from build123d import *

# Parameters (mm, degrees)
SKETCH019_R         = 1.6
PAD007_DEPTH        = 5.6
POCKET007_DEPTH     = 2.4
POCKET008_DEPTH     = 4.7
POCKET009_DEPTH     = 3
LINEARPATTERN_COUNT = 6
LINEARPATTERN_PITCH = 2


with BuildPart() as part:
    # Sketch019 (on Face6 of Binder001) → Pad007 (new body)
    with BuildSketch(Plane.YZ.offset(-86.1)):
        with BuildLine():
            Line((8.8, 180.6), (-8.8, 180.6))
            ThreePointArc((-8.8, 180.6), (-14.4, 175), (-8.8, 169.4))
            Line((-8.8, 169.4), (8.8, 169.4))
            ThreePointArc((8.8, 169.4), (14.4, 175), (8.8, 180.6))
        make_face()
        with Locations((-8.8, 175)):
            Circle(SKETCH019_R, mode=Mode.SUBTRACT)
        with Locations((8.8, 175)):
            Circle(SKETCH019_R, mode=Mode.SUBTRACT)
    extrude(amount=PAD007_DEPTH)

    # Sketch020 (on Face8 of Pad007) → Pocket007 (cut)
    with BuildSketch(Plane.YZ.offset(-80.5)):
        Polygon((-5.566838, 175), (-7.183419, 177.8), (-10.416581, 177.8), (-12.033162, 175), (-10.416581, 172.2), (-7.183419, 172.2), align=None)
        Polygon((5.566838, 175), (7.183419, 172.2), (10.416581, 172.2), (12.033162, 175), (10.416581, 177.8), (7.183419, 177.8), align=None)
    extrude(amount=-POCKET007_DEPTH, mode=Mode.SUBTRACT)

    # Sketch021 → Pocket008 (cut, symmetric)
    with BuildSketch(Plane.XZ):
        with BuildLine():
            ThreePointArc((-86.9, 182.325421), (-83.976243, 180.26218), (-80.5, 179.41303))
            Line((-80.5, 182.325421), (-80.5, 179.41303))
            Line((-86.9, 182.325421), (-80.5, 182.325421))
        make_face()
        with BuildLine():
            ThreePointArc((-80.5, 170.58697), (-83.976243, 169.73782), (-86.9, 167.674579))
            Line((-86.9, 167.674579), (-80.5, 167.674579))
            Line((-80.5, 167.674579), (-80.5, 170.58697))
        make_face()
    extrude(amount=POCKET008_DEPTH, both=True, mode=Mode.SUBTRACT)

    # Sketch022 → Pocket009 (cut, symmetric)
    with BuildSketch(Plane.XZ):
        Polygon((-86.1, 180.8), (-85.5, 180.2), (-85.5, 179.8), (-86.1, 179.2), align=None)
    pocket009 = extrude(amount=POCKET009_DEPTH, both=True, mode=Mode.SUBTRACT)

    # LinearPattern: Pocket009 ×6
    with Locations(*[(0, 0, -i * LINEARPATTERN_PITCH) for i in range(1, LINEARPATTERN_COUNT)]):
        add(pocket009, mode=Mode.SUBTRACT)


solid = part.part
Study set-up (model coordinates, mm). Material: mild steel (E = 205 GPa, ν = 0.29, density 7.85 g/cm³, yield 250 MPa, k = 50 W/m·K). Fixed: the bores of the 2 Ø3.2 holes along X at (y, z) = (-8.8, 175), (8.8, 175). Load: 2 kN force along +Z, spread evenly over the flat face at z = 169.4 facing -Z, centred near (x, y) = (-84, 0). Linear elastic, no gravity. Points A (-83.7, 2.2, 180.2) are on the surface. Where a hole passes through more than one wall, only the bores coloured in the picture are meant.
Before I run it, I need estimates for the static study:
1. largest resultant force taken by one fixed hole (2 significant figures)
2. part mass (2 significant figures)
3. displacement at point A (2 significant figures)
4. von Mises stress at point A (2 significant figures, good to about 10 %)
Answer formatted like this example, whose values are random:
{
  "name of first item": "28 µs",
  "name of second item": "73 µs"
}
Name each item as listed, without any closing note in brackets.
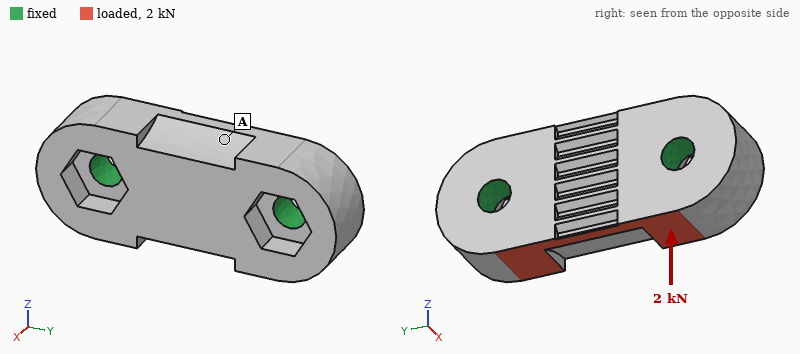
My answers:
{
  "largest resultant force taken by one fixed hole": "1.0 kN",
  "part mass": "11 g",
  "displacement at point A": "1.5 µm",
  "von Mises stress at point A": "21 MPa"
}
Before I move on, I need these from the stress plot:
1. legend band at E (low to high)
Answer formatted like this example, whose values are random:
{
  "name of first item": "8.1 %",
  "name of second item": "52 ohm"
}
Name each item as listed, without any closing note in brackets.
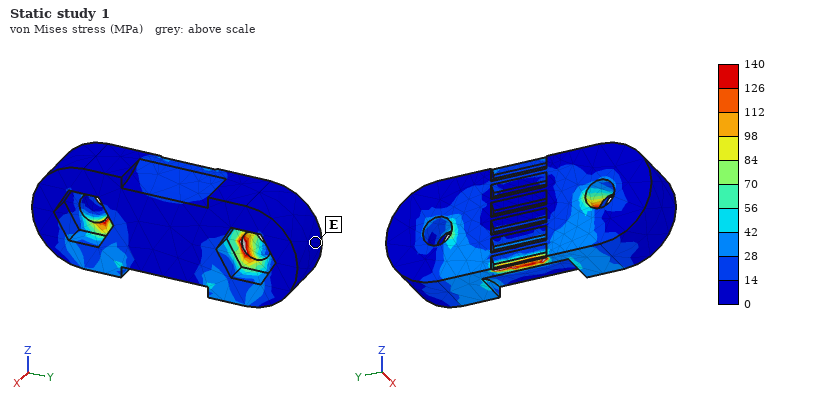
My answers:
{
  "legend band at E": "0 to 14 MPa"
}
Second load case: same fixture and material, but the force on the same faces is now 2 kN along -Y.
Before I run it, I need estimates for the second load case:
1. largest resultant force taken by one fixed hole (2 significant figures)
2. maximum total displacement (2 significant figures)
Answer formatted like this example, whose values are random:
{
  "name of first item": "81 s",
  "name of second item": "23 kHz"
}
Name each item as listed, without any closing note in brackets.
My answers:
{
  "largest resultant force taken by one fixed hole": "1.1 kN",
  "maximum total displacement": "2.7 µm"
}
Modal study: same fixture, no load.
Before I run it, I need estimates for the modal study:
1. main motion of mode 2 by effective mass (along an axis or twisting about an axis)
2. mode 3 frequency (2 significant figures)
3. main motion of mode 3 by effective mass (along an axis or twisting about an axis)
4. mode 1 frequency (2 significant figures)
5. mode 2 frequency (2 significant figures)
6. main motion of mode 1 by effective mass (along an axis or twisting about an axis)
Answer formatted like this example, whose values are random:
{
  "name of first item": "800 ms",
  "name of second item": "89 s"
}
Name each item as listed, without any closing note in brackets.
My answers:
{
  "main motion of mode 2 by effective mass": "along X",
  "mode 3 frequency": "63 kHz",
  "main motion of mode 3 by effective mass": "along Z",
  "mode 1 frequency": "44 kHz",
  "mode 2 frequency": "51 kHz",
  "main motion of mode 1 by effective mass": "along Z"
}
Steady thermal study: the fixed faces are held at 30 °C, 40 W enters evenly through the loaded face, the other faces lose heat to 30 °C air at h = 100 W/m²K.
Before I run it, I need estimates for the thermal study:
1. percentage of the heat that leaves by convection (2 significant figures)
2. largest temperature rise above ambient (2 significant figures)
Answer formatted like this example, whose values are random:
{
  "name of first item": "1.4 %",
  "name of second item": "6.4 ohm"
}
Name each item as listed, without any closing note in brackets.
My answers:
{
  "percentage of the heat that leaves by convection": "5.0 %",
  "largest temperature rise above ambient": "72 K"
}
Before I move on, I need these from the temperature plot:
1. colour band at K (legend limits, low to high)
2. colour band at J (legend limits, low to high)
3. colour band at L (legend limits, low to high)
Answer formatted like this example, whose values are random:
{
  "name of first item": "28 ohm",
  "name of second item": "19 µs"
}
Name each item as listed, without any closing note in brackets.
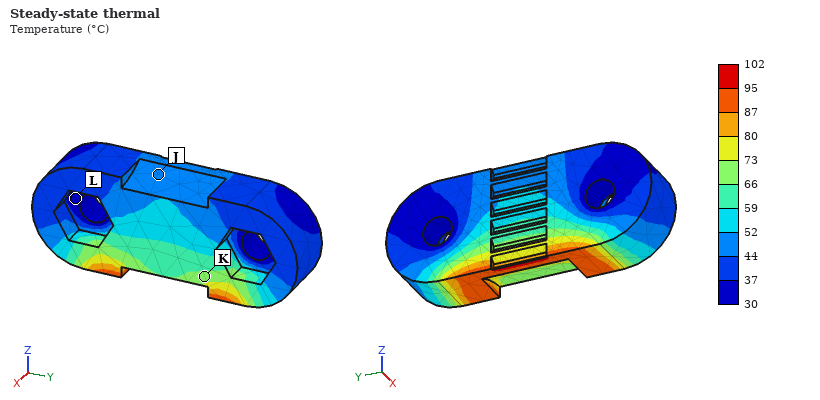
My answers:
{
  "colour band at K": "66 to 73 °C",
  "colour band at J": "44 to 52 °C",
  "colour band at L": "30 to 37 °C"
}
